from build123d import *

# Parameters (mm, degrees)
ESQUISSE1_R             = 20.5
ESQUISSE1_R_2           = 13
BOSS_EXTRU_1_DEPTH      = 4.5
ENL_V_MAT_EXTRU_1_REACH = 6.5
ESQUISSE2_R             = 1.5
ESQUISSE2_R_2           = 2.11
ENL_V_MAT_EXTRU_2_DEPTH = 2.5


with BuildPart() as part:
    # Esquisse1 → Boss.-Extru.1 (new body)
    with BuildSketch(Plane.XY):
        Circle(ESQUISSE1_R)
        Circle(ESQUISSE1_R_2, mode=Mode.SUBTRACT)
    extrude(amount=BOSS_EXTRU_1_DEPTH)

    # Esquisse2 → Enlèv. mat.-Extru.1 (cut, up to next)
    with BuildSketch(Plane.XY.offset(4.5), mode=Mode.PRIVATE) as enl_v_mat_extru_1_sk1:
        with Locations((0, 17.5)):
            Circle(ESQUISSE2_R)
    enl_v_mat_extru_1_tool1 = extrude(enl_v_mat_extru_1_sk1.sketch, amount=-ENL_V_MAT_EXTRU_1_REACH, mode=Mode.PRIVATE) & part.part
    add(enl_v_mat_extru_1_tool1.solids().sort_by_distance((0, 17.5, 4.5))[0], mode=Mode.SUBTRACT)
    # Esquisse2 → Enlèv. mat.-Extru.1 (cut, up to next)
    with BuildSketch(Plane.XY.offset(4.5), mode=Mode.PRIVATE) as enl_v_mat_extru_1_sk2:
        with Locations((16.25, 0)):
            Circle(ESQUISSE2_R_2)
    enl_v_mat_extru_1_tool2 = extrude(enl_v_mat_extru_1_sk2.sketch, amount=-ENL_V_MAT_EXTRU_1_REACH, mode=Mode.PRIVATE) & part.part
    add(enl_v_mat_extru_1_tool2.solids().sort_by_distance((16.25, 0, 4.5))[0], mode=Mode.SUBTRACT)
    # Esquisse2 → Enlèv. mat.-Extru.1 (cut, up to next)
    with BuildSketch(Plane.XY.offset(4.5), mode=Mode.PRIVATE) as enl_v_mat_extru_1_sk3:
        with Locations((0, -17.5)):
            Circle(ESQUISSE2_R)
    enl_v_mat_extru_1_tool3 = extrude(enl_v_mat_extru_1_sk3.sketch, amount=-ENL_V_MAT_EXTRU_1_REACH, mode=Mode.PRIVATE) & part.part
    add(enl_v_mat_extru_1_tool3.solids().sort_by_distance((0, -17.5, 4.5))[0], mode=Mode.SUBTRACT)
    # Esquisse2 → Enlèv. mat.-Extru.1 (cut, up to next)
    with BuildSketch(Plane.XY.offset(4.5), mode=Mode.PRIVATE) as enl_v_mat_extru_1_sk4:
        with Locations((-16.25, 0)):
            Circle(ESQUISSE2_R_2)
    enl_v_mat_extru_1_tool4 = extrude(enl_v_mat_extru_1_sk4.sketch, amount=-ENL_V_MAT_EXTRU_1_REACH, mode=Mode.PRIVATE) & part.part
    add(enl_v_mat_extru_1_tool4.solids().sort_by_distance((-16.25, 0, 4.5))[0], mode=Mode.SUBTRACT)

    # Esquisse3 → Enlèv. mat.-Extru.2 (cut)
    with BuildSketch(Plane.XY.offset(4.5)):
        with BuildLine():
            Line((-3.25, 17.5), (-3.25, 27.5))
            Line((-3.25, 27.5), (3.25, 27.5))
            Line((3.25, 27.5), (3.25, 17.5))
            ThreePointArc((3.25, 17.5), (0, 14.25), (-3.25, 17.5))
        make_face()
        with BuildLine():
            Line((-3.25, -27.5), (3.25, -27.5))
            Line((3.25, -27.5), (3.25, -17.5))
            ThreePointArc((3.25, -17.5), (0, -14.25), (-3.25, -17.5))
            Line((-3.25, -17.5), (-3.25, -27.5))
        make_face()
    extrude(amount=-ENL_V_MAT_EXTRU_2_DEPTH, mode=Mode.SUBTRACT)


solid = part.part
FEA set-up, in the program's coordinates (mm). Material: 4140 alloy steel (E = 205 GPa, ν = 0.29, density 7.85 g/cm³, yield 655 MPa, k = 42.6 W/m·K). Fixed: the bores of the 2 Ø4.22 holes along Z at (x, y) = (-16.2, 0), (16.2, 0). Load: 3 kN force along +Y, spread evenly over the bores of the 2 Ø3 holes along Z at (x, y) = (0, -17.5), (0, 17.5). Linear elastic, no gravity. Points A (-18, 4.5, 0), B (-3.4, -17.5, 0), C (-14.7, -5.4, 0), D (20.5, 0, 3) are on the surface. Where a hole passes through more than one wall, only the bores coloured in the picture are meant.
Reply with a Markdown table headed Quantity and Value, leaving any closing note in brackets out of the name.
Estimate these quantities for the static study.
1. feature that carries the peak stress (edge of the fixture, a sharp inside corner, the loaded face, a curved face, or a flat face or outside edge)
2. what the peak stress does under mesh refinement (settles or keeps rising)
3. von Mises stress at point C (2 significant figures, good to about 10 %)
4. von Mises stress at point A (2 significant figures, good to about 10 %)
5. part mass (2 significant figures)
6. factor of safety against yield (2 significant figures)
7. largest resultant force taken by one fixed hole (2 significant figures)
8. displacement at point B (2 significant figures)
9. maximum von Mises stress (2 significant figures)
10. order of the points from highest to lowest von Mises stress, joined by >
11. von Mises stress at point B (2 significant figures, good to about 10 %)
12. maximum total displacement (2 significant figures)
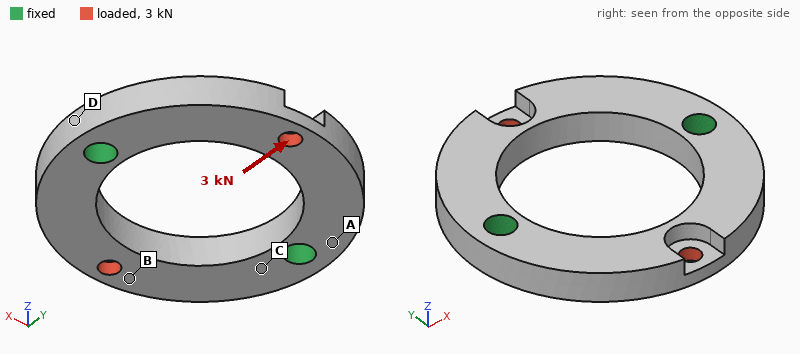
| Quantity | Value |
|---|---|
| feature that carries the peak stress | the loaded face |
| what the peak stress does under mesh refinement | settles |
| von Mises stress at point C | 85 MPa |
| von Mises stress at point A | 50 MPa |
| part mass | 25 g |
| factor of safety against yield | 1.8 |
| largest resultant force taken by one fixed hole | 1.5 kN |
| displacement at point B | 23 µm |
| maximum von Mises stress | 360 MPa |
| order of the points from highest to lowest von Mises stress, joined by > | B > C > A > D |
| von Mises stress at point B | 110 MPa |
| maximum total displacement | 31 µm |
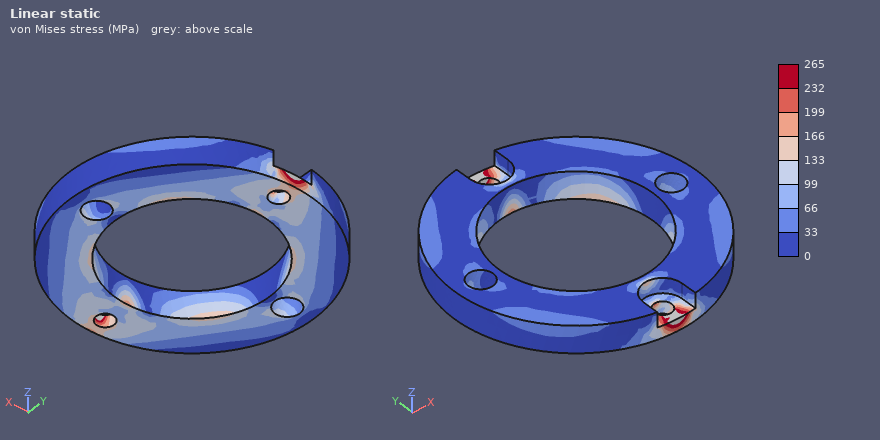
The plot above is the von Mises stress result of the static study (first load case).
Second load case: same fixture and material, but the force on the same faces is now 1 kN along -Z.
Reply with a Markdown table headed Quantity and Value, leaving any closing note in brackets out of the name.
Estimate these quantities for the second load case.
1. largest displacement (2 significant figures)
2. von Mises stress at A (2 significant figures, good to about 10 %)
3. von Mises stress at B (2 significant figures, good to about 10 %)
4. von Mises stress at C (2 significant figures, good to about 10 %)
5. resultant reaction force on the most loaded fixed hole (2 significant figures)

| Quantity | Value |
|---|---|
| largest displacement | 71 µm |
| von Mises stress at A | 120 MPa |
| von Mises stress at B | 48 MPa |
| von Mises stress at C | 150 MPa |
| resultant reaction force on the most loaded fixed hole | 500 N |
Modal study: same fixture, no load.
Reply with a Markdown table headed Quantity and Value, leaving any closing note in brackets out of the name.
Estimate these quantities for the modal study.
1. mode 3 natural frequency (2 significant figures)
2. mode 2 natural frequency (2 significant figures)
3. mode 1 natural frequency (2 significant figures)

| Quantity | Value |
|---|---|
| mode 3 natural frequency | 17 kHz |
| mode 2 natural frequency | 7800 Hz |
| mode 1 natural frequency | 7800 Hz |
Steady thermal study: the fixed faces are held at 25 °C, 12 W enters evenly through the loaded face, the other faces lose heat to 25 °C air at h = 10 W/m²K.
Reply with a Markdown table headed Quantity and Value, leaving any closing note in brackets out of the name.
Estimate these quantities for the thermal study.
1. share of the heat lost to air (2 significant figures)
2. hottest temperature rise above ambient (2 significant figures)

| Quantity | Value |
|---|---|
| share of the heat lost to air | 5.0 % |
| hottest temperature rise above ambient | 65 K |
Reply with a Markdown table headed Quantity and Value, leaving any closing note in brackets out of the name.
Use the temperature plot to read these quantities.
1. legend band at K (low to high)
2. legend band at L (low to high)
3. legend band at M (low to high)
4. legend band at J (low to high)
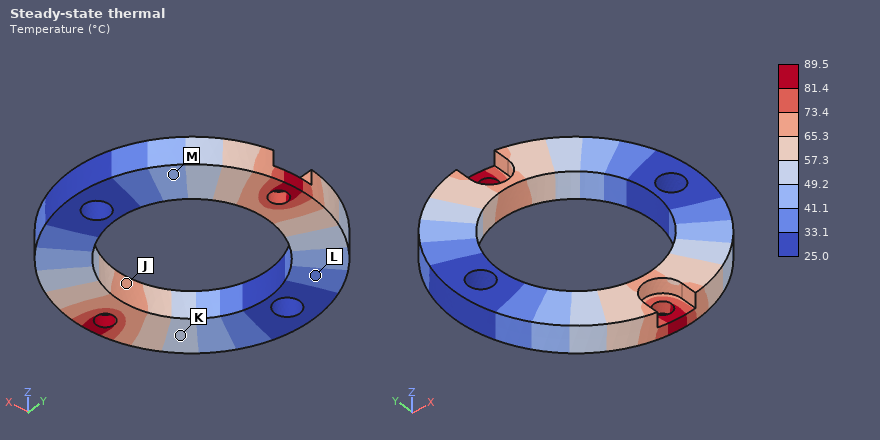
| Quantity | Value |
|---|---|
| legend band at K | 49.2 to 57.3 °C |
| legend band at L | 33.1 to 41.1 °C |
| legend band at M | 41.1 to 49.2 °C |
| legend band at J | 65.3 to 73.4 °C |
